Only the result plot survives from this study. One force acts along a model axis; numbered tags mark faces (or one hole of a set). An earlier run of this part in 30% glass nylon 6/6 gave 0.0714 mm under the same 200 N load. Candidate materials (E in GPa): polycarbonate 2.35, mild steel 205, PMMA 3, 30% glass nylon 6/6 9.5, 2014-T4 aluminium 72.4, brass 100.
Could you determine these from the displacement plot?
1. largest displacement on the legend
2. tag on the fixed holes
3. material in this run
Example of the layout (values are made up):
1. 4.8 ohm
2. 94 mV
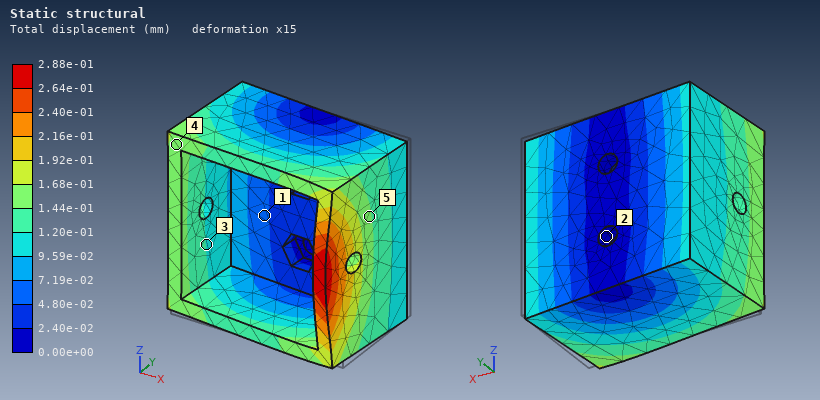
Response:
1. 2.88e-01 mm
2. 2
3. polycarbonate
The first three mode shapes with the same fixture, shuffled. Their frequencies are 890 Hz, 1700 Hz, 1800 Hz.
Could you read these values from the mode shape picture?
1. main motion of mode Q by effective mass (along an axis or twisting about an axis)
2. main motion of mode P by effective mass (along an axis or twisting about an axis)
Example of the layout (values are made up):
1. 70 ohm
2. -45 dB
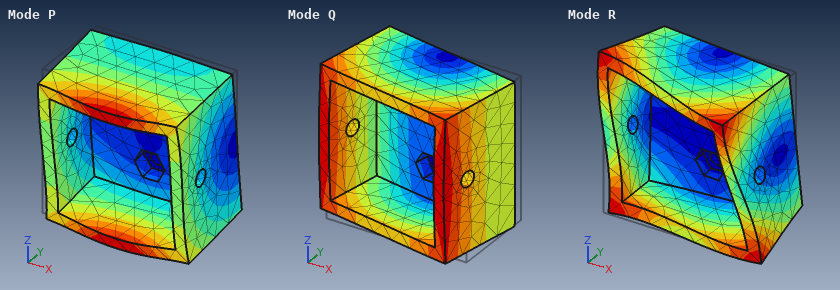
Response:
1. along X
2. along Z
